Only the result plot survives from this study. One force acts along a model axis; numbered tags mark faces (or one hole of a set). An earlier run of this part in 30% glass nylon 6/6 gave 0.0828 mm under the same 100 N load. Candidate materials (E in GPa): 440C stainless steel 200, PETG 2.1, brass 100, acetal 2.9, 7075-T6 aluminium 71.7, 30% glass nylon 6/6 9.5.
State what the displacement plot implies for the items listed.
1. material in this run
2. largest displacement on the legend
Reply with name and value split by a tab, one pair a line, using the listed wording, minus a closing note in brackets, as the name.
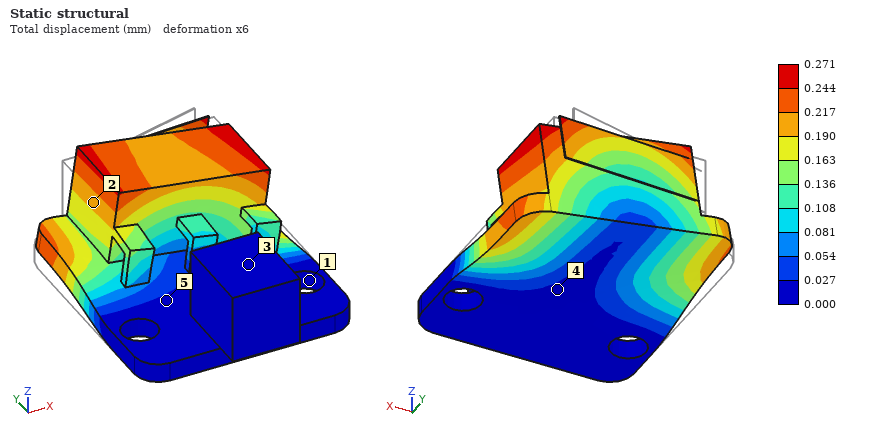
material in this run	acetal
largest displacement on the legend	0.271 mm
